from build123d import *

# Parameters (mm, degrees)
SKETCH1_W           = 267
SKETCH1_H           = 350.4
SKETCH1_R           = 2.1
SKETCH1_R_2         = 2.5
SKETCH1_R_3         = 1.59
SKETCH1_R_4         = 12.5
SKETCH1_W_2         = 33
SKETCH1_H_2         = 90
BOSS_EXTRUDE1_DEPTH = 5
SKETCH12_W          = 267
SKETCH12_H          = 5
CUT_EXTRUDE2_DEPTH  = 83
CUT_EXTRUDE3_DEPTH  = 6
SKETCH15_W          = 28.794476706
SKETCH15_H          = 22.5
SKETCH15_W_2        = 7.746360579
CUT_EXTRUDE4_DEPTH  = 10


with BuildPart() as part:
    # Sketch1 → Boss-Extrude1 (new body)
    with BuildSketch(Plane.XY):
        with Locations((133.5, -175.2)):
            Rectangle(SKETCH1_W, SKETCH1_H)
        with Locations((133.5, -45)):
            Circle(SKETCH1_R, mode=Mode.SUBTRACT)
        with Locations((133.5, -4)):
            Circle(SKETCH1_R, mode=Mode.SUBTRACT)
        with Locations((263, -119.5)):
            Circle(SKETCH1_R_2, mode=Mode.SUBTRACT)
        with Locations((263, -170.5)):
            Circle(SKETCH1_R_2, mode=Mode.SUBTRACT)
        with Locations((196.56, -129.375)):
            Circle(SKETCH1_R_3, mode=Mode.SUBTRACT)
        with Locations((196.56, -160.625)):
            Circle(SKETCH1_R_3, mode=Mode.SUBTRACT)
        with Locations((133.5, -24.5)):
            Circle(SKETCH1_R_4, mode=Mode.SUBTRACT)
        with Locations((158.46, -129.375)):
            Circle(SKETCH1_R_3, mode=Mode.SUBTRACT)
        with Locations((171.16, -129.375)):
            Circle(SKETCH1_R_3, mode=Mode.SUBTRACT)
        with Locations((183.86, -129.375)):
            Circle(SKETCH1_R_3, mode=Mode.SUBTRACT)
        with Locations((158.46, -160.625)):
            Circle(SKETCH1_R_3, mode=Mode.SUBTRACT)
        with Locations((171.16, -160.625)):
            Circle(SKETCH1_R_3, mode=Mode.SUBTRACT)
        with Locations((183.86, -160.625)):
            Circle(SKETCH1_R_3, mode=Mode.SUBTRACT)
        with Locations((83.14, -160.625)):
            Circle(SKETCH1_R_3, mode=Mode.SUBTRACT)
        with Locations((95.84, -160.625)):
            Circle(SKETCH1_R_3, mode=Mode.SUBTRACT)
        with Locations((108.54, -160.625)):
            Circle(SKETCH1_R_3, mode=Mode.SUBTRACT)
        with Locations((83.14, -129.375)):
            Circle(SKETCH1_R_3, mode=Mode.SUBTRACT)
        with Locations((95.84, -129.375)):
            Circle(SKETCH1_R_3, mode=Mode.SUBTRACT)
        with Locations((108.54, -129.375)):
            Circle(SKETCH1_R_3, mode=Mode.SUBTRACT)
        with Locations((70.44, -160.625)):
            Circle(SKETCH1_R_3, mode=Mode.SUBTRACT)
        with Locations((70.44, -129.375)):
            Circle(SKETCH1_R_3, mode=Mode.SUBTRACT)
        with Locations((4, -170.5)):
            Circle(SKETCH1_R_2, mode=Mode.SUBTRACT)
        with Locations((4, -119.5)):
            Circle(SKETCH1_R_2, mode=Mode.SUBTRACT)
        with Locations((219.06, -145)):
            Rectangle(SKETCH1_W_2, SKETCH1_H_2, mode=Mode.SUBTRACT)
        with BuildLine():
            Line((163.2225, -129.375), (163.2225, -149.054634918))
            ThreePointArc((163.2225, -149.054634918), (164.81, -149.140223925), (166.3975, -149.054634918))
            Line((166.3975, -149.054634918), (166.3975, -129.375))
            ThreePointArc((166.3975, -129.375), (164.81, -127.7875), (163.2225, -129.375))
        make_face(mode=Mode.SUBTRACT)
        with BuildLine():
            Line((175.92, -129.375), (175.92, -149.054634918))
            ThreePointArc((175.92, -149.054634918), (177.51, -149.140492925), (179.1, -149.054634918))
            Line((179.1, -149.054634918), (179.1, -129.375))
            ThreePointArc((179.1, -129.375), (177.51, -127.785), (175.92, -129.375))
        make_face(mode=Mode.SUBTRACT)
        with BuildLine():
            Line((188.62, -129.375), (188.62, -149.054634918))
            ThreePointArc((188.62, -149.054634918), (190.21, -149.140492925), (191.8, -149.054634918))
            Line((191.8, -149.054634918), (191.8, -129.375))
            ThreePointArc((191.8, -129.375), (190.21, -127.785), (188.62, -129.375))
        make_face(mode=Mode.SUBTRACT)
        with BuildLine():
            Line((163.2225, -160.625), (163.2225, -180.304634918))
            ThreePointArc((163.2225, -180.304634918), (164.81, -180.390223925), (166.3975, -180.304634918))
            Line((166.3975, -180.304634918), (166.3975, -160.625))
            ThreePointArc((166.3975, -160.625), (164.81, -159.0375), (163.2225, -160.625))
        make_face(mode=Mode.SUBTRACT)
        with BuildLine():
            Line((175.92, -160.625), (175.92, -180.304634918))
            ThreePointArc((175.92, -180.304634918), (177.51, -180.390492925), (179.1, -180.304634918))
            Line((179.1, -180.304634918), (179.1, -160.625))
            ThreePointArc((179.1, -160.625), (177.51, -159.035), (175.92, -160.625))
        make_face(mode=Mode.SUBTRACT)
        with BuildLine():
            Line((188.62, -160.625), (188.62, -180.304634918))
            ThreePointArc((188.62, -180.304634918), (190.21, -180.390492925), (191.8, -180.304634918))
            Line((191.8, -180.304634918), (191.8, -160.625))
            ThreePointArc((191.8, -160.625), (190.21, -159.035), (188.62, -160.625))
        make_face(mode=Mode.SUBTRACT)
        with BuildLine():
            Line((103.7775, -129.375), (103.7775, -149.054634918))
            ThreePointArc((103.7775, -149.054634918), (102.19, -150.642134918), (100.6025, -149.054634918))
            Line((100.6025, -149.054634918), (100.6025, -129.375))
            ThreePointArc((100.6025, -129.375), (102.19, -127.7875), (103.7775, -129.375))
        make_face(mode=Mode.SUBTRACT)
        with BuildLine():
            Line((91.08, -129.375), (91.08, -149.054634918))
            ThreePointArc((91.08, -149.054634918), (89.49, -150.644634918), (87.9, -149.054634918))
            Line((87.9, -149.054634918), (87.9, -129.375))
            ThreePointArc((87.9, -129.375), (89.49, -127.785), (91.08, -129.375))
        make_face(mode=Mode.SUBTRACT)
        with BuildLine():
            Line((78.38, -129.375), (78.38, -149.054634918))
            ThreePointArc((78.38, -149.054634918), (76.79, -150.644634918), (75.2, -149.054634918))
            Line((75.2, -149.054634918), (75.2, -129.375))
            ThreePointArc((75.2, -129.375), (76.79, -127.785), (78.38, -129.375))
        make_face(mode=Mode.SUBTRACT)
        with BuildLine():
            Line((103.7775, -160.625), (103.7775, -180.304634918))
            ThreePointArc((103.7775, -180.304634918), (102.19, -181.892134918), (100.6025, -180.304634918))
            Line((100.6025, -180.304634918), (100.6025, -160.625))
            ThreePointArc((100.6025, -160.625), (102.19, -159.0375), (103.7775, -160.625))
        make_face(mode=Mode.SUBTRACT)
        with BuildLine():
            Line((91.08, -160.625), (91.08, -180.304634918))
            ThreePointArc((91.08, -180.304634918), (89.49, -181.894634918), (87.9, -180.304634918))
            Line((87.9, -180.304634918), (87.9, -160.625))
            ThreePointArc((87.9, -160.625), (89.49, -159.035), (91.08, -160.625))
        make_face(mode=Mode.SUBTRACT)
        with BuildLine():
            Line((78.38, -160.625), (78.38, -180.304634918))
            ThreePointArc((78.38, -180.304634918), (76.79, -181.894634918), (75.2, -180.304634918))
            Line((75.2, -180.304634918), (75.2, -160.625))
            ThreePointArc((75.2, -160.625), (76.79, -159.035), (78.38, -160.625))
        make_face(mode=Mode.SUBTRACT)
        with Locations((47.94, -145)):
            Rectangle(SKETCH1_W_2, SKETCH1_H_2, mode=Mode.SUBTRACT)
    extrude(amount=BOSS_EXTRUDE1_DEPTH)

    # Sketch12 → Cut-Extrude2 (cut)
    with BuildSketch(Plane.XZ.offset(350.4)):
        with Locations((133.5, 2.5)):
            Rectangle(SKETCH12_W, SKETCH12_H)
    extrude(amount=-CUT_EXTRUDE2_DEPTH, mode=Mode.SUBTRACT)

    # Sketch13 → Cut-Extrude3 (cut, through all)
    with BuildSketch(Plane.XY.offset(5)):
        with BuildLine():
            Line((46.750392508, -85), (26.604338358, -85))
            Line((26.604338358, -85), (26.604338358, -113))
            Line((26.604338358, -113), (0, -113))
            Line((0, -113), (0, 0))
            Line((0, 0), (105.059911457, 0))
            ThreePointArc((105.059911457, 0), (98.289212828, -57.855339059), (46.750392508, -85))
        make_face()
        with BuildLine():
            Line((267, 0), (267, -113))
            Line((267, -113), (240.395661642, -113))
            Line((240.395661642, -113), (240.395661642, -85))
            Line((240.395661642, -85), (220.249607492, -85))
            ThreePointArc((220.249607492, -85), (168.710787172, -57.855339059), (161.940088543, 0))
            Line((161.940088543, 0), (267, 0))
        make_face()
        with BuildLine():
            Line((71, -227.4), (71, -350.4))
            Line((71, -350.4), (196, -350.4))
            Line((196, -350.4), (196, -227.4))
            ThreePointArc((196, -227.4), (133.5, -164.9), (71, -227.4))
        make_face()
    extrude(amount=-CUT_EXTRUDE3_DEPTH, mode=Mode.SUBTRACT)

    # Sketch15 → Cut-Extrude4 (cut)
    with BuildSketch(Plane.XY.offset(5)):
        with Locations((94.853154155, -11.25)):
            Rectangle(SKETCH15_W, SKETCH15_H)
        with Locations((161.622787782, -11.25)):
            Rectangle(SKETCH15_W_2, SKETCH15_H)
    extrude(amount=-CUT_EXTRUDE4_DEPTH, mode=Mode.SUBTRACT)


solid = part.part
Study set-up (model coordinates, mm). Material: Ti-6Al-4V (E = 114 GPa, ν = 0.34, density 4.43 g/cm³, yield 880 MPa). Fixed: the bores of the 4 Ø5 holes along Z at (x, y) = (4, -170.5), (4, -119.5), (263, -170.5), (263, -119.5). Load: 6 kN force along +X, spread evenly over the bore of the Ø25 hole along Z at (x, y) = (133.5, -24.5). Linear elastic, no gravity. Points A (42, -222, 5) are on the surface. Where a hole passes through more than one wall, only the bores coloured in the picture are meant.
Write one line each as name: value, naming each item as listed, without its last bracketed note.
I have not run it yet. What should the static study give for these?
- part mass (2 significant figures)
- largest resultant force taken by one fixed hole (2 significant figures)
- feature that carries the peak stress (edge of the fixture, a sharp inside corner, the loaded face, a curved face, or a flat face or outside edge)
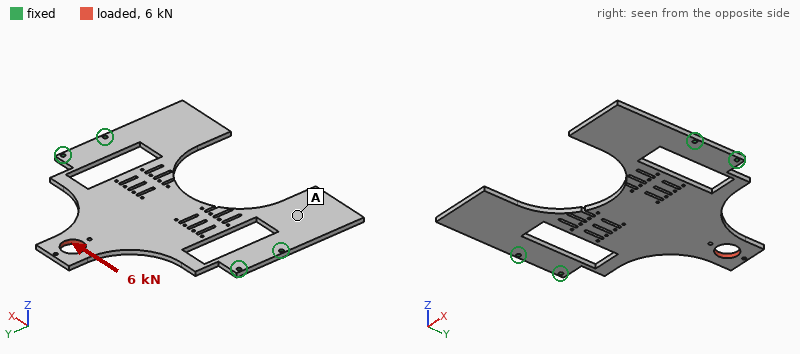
part mass: 760 g
largest resultant force taken by one fixed hole: 2.8 kN
feature that carries the peak stress: a flat face or outside edge
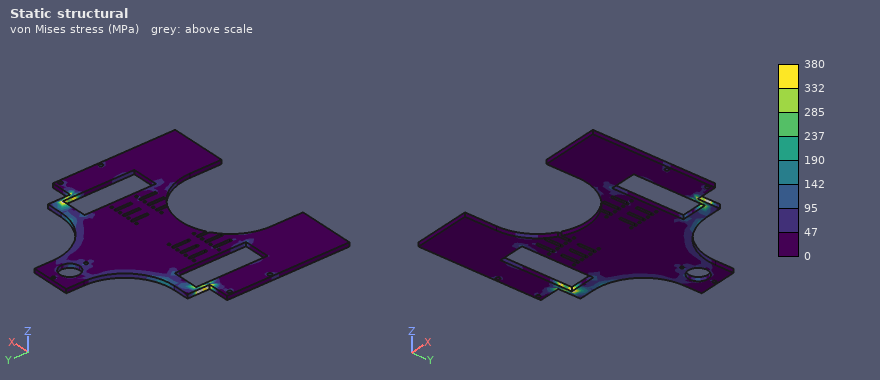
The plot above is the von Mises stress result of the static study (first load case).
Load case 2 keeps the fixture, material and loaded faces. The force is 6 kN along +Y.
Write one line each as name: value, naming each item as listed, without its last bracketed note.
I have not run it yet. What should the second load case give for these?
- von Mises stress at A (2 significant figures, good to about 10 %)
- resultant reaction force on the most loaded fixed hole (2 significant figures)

von Mises stress at A: 11 MPa
resultant reaction force on the most loaded fixed hole: 3.2 kN
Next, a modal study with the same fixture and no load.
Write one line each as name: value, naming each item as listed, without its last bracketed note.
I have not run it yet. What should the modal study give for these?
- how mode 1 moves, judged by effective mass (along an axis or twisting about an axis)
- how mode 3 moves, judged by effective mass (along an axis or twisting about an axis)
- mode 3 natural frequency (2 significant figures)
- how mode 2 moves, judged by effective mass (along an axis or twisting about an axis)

how mode 1 moves, judged by effective mass: along Z
how mode 3 moves, judged by effective mass: twisting about Y
mode 3 natural frequency: 310 Hz
how mode 2 moves, judged by effective mass: along Z
